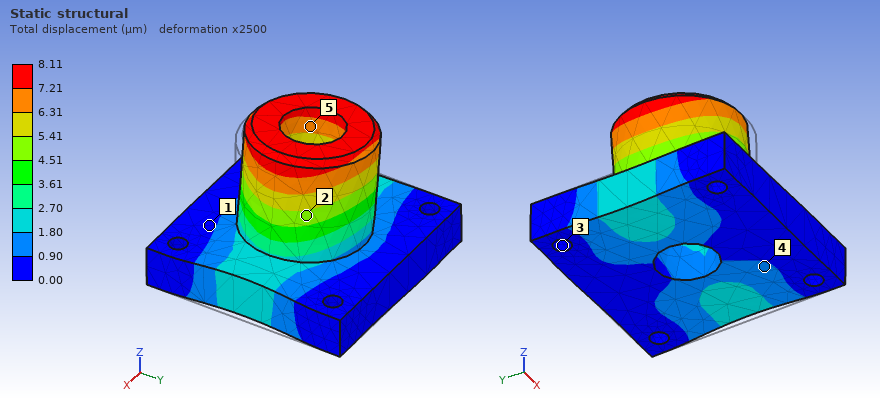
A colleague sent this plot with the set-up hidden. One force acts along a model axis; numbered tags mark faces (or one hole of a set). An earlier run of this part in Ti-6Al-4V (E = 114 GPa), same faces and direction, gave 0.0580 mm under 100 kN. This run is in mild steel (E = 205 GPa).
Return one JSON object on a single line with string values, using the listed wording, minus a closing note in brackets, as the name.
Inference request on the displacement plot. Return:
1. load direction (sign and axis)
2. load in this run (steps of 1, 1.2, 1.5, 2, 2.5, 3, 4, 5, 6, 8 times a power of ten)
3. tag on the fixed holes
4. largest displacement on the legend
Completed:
{"load direction": "-X", "load in this run": "25 kN", "tag on the fixed holes": "3", "largest displacement on the legend": "8.11 µm"}
